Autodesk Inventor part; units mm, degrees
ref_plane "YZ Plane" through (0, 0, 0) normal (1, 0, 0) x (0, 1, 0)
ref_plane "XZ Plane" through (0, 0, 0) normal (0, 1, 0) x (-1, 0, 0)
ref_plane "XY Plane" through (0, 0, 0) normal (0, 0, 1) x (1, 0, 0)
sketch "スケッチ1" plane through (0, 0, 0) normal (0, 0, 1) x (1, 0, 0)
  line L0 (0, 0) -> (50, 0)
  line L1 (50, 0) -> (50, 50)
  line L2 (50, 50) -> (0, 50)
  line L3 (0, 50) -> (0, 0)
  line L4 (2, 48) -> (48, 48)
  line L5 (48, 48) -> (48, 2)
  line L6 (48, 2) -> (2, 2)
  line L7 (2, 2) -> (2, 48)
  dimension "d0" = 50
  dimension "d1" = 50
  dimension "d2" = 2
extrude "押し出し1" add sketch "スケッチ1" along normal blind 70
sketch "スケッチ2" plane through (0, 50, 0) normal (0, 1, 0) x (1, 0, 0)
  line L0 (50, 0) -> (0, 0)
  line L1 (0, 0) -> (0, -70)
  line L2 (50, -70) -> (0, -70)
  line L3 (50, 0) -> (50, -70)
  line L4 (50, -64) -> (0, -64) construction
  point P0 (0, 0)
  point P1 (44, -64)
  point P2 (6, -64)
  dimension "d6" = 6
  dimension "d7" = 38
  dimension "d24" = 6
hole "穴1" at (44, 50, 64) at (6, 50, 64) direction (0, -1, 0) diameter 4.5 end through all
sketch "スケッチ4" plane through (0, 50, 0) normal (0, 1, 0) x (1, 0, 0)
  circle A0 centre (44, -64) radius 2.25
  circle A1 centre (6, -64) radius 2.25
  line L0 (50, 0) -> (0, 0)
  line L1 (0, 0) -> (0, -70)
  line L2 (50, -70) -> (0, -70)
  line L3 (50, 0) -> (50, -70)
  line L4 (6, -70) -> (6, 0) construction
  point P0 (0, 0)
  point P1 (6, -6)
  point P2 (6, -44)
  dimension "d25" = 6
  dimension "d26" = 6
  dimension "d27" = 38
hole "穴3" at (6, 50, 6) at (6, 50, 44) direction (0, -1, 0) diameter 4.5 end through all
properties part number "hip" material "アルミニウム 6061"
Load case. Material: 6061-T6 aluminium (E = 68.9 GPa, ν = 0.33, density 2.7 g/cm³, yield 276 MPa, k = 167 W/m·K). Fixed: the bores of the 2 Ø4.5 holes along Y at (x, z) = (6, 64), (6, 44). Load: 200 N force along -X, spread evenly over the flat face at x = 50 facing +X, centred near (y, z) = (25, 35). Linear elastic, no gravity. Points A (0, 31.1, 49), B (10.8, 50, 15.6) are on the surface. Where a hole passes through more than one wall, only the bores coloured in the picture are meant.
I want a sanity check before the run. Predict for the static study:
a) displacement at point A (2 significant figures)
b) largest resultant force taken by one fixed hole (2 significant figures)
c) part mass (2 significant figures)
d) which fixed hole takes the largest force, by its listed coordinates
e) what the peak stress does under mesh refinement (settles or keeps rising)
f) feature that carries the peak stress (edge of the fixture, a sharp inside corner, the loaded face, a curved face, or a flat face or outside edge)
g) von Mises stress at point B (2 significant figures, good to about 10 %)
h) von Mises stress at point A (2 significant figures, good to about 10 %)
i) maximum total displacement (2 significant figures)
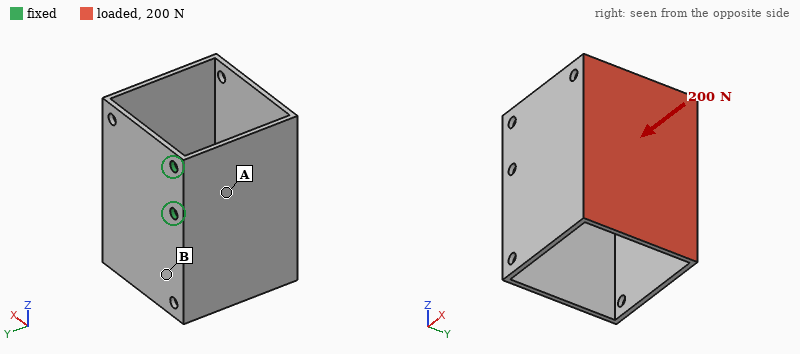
0.23 mm
260 N
72 g
(6, 44)
keeps rising
edge of the fixture
12 MPa
31 MPa
1.1 mm
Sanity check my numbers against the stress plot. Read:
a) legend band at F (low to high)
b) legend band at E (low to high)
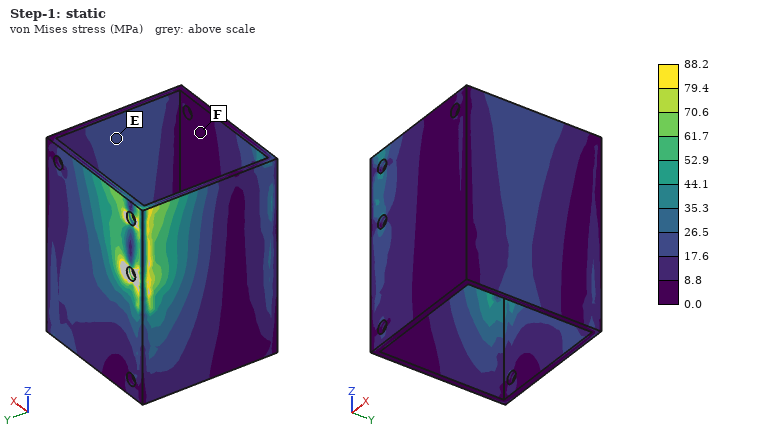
0.0 to 8.8 MPa
17.6 to 26.5 MPa
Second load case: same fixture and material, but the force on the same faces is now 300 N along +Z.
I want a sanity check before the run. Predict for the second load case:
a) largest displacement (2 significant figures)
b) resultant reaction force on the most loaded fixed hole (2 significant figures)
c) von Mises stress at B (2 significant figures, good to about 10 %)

0.56 mm
680 N
23 MPa
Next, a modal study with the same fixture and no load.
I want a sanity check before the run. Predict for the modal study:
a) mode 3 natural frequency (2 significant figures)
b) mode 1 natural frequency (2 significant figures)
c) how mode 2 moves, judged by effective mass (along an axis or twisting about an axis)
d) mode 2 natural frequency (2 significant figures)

800 Hz
260 Hz
along Z
660 Hz
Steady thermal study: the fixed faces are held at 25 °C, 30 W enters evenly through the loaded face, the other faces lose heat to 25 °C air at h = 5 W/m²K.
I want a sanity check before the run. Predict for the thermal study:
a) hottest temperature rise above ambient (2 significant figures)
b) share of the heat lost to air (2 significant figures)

57 K
14 %
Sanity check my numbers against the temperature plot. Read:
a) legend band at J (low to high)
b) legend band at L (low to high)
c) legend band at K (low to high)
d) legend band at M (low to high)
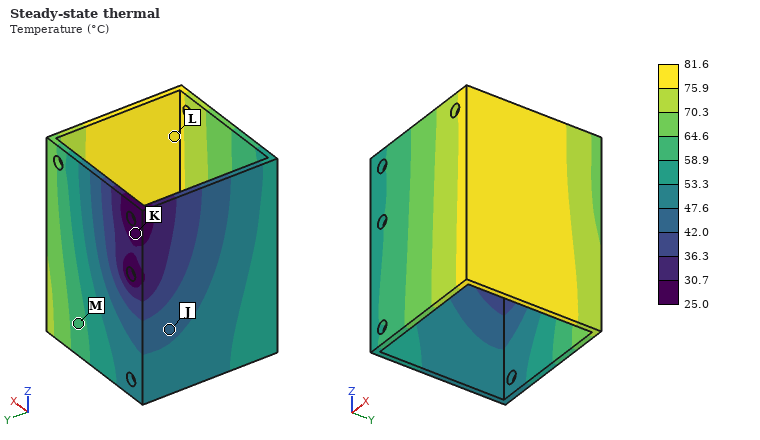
42.0 to 47.6 °C
75.9 to 81.6 °C
25.0 to 30.7 °C
58.9 to 64.6 °C
